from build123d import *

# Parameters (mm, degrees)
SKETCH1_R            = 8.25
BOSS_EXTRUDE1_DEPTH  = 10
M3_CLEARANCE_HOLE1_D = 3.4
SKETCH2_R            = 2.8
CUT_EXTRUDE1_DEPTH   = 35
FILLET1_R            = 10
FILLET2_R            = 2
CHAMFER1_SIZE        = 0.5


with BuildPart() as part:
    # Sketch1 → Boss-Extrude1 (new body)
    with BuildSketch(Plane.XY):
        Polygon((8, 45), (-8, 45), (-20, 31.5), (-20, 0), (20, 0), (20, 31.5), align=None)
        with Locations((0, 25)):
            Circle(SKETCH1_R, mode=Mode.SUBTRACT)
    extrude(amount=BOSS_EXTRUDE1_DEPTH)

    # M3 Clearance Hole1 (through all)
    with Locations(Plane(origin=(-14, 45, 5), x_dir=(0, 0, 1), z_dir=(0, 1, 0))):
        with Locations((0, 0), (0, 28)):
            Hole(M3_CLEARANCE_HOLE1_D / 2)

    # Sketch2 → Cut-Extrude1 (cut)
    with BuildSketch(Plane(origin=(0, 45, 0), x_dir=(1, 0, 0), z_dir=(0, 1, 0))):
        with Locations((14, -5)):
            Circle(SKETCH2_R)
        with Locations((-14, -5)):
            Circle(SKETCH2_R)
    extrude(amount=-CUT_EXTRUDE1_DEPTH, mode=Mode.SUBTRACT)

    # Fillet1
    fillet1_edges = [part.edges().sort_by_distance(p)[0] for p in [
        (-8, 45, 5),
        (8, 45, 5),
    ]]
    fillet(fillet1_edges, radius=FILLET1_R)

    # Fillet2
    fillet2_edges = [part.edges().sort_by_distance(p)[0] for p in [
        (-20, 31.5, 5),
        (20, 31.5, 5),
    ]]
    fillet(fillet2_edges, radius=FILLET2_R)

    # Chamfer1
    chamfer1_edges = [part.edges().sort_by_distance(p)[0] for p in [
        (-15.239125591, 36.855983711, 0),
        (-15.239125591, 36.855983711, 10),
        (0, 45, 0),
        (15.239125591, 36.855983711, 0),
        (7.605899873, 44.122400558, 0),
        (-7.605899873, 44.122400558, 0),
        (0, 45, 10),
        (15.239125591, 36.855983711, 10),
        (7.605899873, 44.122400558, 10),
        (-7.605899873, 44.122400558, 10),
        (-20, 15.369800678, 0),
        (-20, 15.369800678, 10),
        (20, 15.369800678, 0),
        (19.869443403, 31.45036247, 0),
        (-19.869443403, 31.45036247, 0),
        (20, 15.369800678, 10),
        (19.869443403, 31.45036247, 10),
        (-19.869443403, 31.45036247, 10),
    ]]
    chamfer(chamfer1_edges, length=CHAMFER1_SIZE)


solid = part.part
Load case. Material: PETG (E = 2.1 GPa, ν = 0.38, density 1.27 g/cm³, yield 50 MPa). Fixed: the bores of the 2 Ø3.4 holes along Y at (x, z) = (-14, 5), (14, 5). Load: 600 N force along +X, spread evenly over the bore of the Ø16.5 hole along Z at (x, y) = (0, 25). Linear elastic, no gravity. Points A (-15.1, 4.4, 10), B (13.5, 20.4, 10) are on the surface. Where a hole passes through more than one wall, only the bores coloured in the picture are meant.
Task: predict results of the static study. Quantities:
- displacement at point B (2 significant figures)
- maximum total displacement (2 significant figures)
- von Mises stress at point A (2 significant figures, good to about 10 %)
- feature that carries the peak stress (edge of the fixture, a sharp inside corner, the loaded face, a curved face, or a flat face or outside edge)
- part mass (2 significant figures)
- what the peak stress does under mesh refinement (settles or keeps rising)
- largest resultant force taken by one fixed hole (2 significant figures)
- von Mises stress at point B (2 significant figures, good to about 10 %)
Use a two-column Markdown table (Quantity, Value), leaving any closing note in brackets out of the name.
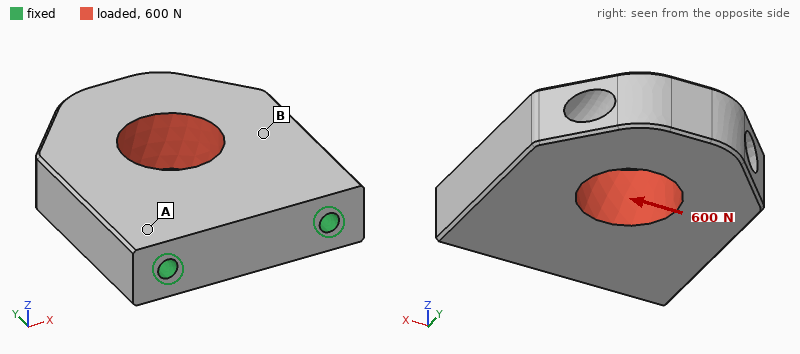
| Quantity | Value |
|---|---|
| displacement at point B | 0.071 mm |
| maximum total displacement | 0.17 mm |
| von Mises stress at point A | 1.6 MPa |
| feature that carries the peak stress | edge of the fixture |
| part mass | 16 g |
| what the peak stress does under mesh refinement | keeps rising |
| largest resultant force taken by one fixed hole | 460 N |
| von Mises stress at point B | 5.9 MPa |
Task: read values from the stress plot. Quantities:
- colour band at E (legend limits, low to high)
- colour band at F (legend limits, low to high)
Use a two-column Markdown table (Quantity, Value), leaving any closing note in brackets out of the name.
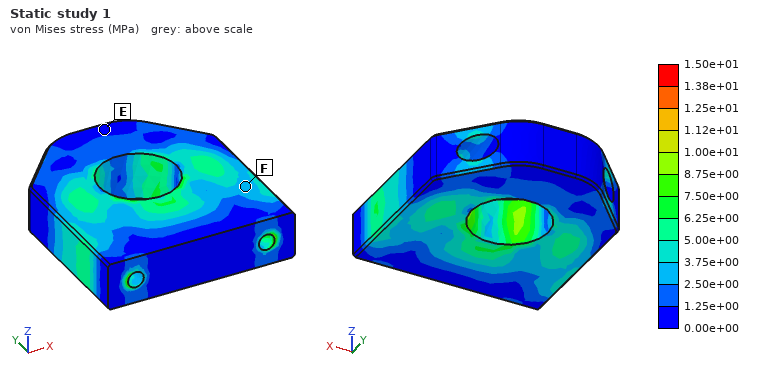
| Quantity | Value |
|---|---|
| colour band at E | 0.00e+00 to 1.25e+00 MPa |
| colour band at F | 2.50e+00 to 3.75e+00 MPa |
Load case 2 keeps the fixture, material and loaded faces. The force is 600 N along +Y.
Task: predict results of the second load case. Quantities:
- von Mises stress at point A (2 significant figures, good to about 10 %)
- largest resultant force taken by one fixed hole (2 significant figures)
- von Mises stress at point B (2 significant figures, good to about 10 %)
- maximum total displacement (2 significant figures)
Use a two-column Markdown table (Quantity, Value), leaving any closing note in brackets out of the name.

| Quantity | Value |
|---|---|
| von Mises stress at point A | 0.81 MPa |
| largest resultant force taken by one fixed hole | 310 N |
| von Mises stress at point B | 2.8 MPa |
| maximum total displacement | 47 µm |
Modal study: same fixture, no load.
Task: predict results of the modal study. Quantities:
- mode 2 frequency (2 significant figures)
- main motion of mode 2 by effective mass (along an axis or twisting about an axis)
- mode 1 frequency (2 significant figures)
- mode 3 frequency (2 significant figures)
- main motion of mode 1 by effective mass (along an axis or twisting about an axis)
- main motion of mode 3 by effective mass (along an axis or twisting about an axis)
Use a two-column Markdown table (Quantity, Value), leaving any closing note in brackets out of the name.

| Quantity | Value |
|---|---|
| mode 2 frequency | 3000 Hz |
| main motion of mode 2 by effective mass | along X |
| mode 1 frequency | 1200 Hz |
| mode 3 frequency | 3300 Hz |
| main motion of mode 1 by effective mass | along Z |
| main motion of mode 3 by effective mass | twisting about Y |
